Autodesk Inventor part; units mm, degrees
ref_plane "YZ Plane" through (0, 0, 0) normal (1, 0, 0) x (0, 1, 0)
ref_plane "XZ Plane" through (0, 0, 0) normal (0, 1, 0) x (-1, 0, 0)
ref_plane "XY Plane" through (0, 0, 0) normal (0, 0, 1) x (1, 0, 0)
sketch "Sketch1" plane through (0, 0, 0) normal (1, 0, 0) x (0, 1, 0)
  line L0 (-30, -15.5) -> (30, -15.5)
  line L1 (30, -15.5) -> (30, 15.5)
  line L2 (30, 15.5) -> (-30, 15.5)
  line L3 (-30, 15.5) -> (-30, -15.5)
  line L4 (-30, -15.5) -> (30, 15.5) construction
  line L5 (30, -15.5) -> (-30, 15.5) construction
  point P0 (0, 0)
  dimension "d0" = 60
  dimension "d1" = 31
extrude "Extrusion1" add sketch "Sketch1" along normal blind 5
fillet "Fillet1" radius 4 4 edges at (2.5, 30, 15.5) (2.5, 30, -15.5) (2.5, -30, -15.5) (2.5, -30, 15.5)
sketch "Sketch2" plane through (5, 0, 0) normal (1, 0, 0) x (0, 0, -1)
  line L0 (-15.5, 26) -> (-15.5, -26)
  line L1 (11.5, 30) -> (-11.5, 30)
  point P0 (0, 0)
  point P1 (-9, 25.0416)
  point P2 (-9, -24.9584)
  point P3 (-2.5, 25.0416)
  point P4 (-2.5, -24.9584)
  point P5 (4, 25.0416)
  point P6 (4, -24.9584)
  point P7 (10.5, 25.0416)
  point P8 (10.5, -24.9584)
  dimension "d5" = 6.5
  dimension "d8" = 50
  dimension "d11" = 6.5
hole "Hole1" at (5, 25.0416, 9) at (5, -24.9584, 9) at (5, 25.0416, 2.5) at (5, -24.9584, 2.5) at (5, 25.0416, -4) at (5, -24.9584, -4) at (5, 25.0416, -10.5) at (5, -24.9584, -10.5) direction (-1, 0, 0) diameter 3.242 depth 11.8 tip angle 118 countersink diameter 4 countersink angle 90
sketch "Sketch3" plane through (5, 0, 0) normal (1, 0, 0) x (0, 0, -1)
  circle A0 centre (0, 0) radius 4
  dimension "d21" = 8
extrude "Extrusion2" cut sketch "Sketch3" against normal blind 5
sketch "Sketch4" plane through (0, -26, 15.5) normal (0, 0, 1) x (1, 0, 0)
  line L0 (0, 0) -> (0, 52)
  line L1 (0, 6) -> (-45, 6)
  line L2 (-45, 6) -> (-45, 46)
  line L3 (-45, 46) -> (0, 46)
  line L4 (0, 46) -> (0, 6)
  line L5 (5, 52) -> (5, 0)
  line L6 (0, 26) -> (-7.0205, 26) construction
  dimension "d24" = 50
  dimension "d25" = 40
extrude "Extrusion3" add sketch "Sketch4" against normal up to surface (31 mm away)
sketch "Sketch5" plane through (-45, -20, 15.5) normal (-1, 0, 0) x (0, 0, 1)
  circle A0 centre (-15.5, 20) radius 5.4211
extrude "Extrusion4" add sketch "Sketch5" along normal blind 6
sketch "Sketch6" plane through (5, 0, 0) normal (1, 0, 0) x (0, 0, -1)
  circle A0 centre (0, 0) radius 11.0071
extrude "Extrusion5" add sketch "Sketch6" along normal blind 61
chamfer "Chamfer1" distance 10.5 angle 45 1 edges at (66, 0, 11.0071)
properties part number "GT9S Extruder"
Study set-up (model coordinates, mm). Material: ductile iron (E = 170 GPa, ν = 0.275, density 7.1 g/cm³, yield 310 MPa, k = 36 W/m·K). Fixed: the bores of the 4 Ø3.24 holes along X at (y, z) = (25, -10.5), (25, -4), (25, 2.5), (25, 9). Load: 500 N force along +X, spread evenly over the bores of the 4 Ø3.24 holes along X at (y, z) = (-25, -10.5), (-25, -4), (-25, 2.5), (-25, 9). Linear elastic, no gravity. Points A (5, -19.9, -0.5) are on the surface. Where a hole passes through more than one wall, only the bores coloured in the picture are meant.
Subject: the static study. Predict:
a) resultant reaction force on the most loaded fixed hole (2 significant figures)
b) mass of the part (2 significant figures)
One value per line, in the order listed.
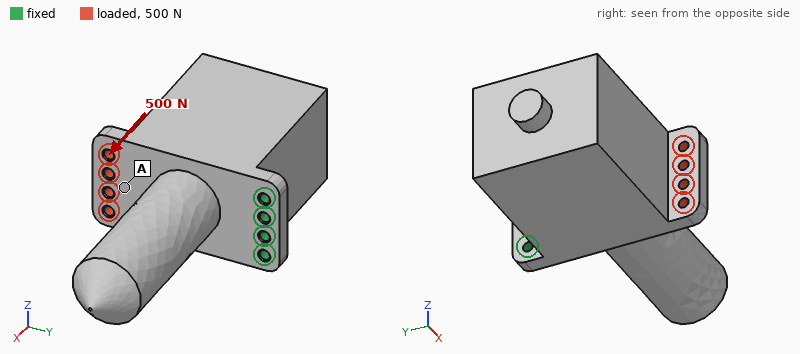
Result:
200 N
610 g
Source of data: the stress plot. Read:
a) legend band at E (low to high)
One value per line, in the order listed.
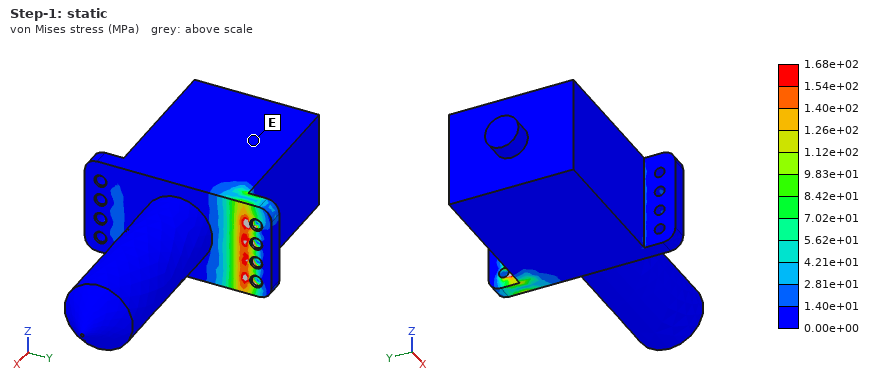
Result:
0.00e+00 to 1.40e+01 MPa
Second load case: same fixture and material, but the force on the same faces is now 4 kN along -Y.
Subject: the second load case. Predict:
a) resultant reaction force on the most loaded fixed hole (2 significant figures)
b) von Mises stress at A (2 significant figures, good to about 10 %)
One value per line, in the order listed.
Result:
1.1 kN
28 MPa
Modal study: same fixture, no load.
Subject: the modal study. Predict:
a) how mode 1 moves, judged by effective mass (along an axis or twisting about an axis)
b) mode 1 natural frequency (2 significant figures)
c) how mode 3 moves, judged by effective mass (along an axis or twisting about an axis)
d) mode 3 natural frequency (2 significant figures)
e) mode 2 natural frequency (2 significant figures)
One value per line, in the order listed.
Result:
along X
480 Hz
along Z
2700 Hz
1500 Hz
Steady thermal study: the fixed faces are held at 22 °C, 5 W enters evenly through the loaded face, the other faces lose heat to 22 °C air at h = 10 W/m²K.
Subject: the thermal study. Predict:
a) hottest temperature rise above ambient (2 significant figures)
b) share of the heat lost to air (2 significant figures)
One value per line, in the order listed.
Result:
21 K
24 %
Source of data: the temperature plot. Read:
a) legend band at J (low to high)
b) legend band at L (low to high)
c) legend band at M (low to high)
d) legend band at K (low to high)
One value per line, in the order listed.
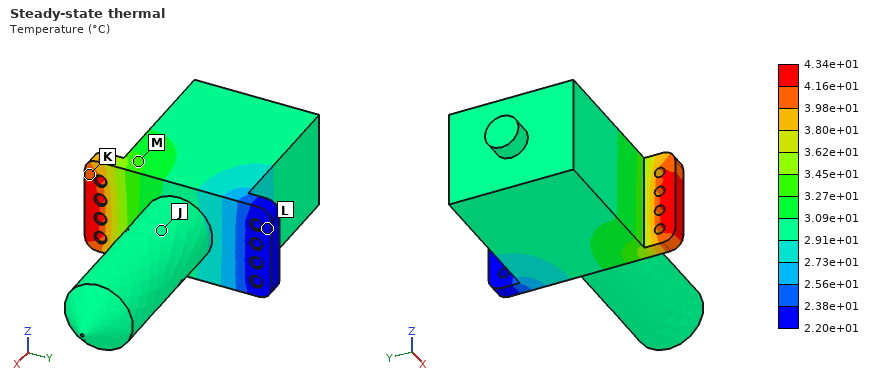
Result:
2.91e+01 to 3.09e+01 °C
2.20e+01 to 2.38e+01 °C
3.27e+01 to 3.45e+01 °C
3.98e+01 to 4.16e+01 °C
